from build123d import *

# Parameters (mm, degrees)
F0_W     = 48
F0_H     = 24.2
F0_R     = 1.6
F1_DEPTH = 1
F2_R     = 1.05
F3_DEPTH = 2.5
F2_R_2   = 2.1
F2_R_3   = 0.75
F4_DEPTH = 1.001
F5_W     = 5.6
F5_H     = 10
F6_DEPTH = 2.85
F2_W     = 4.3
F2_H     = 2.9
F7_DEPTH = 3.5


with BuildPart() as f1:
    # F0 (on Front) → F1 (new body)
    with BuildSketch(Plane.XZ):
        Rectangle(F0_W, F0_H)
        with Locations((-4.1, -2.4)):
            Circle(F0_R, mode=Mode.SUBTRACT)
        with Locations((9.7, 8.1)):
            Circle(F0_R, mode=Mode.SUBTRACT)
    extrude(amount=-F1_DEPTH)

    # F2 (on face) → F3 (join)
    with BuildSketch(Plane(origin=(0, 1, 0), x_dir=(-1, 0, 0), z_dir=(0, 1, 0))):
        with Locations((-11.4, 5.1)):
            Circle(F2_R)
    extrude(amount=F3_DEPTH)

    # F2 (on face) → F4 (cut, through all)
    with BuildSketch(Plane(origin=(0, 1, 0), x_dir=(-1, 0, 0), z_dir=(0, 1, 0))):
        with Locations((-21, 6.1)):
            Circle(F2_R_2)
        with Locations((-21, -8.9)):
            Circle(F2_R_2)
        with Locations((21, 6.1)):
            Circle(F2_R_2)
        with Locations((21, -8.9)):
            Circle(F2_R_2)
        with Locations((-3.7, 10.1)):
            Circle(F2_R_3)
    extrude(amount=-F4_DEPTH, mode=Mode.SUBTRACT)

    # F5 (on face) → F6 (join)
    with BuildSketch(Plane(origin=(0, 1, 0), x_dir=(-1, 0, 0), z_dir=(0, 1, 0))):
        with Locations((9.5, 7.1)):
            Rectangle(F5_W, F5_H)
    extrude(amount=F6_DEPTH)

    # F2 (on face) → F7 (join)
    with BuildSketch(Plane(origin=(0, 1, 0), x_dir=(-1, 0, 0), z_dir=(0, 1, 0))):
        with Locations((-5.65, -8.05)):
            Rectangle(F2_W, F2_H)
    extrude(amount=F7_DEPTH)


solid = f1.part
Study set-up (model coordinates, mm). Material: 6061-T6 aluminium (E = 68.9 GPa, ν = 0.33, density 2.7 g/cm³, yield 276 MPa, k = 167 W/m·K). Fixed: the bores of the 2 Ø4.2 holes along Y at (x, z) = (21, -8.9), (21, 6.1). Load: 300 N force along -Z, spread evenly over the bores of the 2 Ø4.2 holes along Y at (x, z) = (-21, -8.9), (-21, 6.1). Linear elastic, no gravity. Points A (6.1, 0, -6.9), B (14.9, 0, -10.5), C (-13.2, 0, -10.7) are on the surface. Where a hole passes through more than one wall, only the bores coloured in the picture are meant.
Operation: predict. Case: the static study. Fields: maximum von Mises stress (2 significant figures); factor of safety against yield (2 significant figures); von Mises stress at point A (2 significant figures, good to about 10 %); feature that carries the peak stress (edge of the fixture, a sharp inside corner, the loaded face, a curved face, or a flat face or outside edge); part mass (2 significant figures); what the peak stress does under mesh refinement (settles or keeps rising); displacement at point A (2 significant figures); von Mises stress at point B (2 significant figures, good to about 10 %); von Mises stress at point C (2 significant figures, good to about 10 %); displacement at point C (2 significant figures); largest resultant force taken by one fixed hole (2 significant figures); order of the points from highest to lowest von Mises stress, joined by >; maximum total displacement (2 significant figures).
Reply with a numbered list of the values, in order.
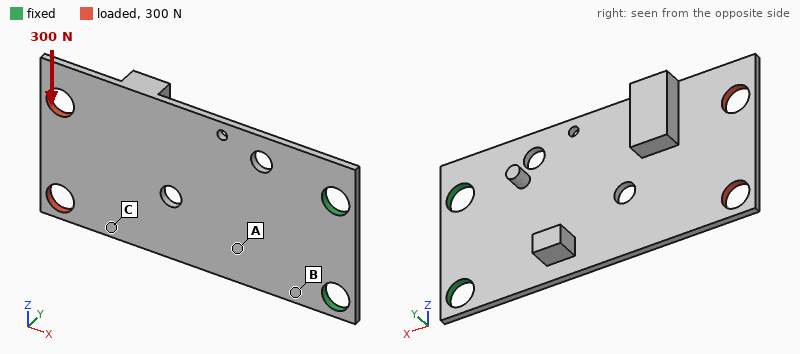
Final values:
1. 230 MPa
2. 1.2
3. 55 MPa
4. a curved face
5. 3.5 g
6. settles
7. 0.028 mm
8. 110 MPa
9. 22 MPa
10. 0.098 mm
11. 750 N
12. B > A > C
13. 0.14 mm
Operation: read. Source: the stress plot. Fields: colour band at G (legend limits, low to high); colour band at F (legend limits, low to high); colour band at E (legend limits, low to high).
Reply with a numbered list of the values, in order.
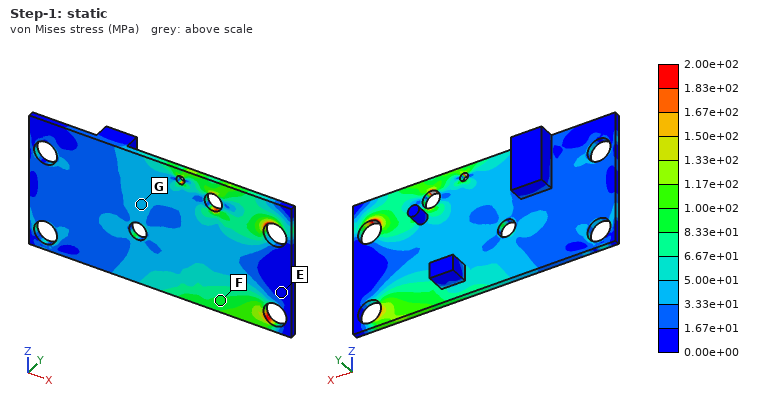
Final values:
1. 3.33e+01 to 5.00e+01 MPa
2. 8.33e+01 to 1.00e+02 MPa
3. 0.00e+00 to 1.67e+01 MPa
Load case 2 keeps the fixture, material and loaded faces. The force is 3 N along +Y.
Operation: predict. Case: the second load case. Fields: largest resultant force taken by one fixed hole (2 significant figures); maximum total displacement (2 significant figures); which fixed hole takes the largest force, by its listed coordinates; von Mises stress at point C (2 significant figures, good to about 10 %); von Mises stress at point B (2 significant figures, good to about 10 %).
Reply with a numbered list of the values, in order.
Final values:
1. 1.7 N
2. 0.52 mm
3. (21, 6.1)
4. 5.6 MPa
5. 29 MPa
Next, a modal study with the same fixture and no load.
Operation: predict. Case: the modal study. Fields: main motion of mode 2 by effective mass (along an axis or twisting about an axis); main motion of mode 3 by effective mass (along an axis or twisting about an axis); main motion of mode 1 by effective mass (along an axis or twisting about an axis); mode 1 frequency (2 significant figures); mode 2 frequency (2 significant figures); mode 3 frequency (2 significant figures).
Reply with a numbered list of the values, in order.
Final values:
1. twisting about X
2. along Y
3. along Y
4. 420 Hz
5. 1600 Hz
6. 2700 Hz
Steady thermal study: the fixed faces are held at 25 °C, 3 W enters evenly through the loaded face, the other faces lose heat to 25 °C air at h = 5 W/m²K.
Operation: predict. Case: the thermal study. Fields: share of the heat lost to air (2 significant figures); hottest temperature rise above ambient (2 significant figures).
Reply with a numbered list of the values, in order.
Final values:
1. 6.2 %
2. 35 K
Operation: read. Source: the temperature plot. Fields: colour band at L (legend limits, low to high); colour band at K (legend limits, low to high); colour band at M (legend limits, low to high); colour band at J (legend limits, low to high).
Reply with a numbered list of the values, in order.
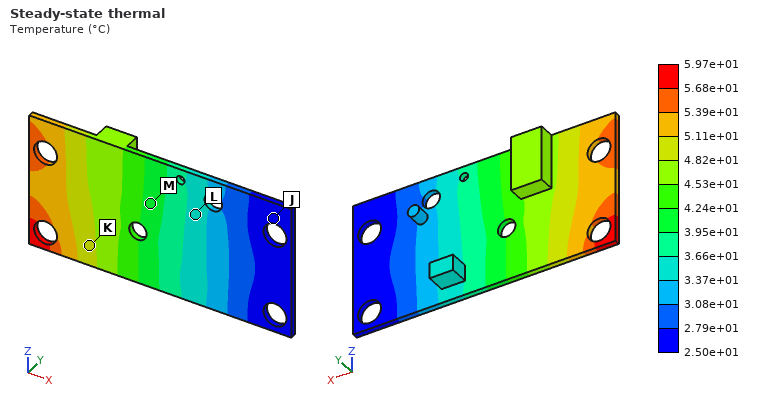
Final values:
1. 3.37e+01 to 3.66e+01 °C
2. 4.82e+01 to 5.11e+01 °C
3. 3.95e+01 to 4.24e+01 °C
4. 2.50e+01 to 2.79e+01 °C
